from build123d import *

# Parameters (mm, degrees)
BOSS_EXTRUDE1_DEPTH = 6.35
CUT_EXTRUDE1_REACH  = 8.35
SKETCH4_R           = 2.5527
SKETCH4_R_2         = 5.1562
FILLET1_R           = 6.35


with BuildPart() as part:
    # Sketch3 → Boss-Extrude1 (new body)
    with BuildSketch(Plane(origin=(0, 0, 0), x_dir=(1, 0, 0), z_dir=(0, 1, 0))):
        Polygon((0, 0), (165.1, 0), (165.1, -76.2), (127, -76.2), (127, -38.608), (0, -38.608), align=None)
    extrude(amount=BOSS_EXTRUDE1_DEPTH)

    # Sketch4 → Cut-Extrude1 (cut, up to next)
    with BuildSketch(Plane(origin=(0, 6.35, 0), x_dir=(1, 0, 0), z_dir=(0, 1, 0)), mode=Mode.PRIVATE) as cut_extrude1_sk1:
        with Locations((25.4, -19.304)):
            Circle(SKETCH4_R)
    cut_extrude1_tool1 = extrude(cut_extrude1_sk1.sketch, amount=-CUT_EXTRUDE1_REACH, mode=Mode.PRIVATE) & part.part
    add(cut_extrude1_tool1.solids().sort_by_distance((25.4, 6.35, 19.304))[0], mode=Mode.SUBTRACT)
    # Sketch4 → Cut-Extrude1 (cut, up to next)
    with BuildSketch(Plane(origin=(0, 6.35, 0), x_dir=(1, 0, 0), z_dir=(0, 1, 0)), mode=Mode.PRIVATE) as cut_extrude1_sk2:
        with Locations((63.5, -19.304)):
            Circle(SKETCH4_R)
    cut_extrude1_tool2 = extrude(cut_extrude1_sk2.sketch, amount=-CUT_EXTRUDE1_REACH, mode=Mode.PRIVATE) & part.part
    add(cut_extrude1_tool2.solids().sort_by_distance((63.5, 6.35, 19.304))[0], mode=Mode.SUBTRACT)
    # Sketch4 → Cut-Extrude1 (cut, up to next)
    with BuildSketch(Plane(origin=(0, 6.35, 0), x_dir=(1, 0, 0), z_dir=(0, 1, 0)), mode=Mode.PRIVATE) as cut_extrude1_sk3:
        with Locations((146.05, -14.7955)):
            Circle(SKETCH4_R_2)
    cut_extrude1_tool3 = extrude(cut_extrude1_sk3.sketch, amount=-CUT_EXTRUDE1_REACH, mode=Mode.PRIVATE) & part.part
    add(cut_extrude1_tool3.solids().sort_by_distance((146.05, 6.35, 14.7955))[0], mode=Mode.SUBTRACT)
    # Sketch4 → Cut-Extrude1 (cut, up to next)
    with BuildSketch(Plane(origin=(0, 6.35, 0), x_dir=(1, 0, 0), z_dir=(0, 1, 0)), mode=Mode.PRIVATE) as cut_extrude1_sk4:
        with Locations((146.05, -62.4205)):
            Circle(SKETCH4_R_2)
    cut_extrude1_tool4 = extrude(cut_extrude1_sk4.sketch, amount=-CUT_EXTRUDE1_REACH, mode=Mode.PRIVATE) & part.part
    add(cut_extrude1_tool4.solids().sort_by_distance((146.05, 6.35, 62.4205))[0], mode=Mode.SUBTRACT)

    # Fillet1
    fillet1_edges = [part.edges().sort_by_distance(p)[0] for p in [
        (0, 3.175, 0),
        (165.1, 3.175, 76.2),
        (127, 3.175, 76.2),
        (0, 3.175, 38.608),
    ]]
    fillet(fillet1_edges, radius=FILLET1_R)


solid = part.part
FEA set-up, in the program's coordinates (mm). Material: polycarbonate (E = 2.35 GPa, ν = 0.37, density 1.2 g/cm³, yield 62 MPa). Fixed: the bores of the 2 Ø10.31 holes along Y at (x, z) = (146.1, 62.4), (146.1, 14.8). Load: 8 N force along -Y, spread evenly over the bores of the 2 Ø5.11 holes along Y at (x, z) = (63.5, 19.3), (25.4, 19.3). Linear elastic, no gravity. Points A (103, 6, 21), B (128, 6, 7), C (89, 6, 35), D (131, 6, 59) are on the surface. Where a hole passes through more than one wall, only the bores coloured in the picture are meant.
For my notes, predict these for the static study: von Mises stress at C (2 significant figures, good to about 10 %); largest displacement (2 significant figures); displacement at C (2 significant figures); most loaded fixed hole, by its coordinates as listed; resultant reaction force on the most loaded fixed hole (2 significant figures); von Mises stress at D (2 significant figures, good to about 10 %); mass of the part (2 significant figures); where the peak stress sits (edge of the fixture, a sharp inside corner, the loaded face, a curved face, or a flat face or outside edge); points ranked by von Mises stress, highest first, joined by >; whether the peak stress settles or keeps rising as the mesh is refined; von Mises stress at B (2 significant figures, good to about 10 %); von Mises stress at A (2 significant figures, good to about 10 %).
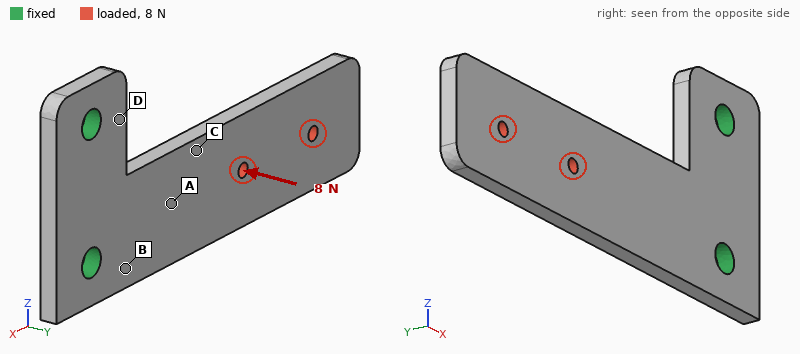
1.4 MPa
2.1 mm
0.45 mm
(146.1, 14.8)
9.6 N
0.51 MPa
58 g
edge of the fixture
B > A > C > D
keeps rising
2.4 MPa
1.7 MPa
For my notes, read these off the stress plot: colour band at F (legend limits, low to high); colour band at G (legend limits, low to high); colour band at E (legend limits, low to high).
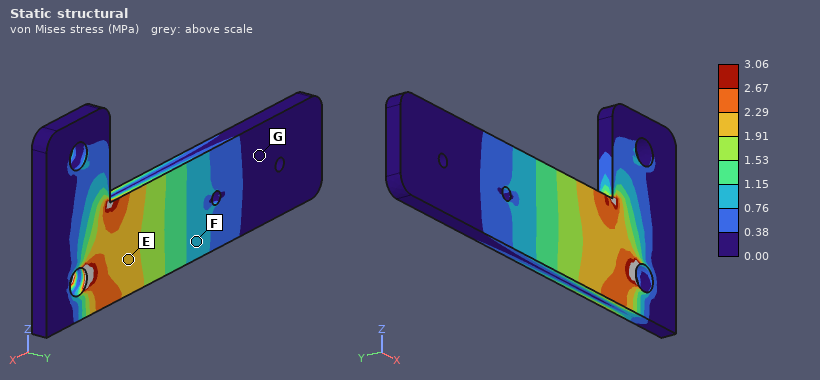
0.76 to 1.15 MPa
0.00 to 0.38 MPa
1.91 to 2.29 MPa
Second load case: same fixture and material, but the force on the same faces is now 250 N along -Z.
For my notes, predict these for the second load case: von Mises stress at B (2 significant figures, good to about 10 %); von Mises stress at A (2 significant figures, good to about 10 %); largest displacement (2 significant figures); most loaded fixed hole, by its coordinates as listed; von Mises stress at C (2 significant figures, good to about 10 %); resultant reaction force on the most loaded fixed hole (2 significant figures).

7.8 MPa
2.8 MPa
2.1 mm
(146.1, 62.4)
5.6 MPa
520 N
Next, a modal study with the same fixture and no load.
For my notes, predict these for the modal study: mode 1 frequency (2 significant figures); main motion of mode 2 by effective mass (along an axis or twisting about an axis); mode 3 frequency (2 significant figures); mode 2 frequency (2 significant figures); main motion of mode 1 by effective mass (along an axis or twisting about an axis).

73 Hz
along Z
440 Hz
400 Hz
along Y
